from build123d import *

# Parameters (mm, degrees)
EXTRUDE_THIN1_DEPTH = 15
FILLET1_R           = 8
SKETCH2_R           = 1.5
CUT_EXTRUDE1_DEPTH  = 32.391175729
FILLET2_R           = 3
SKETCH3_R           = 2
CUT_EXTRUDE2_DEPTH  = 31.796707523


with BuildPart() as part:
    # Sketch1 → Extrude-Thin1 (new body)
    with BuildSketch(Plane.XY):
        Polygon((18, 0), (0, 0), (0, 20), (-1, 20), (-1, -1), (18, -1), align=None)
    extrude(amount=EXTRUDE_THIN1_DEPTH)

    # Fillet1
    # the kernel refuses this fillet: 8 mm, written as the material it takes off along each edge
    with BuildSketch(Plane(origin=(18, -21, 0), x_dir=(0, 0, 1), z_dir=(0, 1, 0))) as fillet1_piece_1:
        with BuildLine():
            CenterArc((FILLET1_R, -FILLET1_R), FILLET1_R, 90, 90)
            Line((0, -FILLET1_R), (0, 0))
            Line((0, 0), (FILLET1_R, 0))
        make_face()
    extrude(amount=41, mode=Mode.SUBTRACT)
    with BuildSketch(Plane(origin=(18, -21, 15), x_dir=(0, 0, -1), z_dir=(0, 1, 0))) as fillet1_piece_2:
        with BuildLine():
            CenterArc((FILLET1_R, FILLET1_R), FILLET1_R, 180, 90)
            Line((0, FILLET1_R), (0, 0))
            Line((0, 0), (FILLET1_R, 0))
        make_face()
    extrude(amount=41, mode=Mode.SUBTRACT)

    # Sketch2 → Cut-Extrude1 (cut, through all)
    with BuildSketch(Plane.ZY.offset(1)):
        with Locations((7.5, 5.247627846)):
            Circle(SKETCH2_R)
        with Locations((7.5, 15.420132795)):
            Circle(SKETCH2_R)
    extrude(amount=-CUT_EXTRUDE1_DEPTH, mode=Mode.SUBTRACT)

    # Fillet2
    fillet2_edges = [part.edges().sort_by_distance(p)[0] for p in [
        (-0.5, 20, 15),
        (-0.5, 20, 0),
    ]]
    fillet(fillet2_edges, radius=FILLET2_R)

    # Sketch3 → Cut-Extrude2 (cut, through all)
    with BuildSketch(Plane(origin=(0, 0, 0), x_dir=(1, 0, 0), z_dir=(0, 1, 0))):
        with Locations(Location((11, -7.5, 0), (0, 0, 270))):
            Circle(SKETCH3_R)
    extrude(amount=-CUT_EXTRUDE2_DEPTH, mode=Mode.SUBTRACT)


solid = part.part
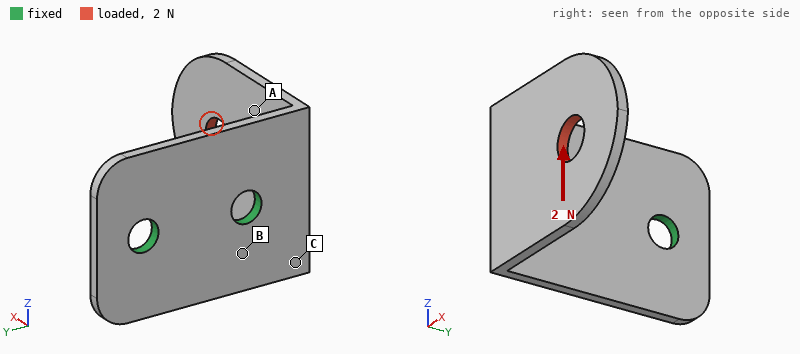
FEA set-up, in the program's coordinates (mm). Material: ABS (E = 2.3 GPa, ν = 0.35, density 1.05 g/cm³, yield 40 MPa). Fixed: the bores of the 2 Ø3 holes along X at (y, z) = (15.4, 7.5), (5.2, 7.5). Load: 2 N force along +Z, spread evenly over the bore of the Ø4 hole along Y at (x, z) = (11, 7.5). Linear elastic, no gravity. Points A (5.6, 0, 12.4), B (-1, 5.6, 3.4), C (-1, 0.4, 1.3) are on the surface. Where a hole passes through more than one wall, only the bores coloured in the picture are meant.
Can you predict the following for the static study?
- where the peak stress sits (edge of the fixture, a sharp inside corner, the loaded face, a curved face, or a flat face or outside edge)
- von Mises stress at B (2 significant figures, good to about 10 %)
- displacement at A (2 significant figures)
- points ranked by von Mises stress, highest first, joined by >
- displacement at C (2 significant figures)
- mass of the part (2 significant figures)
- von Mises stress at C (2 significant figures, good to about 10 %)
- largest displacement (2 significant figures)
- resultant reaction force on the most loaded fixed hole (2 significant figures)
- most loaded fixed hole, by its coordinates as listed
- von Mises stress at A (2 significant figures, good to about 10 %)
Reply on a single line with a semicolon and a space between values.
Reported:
a flat face or outside edge; 4.1 MPa; 0.15 mm; B > C > A; 0.11 mm; 0.55 g; 2.8 MPa; 0.36 mm; 2.7 N; (5.2, 7.5); 1.2 MPa
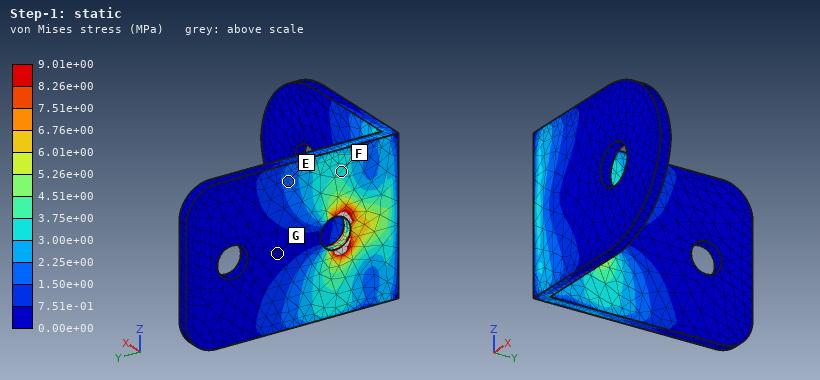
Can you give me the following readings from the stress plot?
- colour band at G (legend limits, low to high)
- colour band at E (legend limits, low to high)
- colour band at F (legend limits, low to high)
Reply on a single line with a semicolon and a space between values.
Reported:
0.00e+00 to 7.51e-01 MPa; 1.50e+00 to 2.25e+00 MPa; 3.00e+00 to 3.75e+00 MPa
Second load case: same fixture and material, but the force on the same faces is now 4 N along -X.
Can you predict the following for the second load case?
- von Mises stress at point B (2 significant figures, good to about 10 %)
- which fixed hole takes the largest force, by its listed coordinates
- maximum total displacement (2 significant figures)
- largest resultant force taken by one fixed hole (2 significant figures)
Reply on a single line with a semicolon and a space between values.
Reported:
2.3 MPa; (5.2, 7.5); 0.35 mm; 4.3 N
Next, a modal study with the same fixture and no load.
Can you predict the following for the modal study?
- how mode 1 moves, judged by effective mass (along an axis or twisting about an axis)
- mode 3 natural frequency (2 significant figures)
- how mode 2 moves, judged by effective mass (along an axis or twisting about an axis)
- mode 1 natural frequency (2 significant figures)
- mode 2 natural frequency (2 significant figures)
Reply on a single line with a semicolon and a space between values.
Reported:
along Y; 2300 Hz; along Z; 600 Hz; 1000 Hz
